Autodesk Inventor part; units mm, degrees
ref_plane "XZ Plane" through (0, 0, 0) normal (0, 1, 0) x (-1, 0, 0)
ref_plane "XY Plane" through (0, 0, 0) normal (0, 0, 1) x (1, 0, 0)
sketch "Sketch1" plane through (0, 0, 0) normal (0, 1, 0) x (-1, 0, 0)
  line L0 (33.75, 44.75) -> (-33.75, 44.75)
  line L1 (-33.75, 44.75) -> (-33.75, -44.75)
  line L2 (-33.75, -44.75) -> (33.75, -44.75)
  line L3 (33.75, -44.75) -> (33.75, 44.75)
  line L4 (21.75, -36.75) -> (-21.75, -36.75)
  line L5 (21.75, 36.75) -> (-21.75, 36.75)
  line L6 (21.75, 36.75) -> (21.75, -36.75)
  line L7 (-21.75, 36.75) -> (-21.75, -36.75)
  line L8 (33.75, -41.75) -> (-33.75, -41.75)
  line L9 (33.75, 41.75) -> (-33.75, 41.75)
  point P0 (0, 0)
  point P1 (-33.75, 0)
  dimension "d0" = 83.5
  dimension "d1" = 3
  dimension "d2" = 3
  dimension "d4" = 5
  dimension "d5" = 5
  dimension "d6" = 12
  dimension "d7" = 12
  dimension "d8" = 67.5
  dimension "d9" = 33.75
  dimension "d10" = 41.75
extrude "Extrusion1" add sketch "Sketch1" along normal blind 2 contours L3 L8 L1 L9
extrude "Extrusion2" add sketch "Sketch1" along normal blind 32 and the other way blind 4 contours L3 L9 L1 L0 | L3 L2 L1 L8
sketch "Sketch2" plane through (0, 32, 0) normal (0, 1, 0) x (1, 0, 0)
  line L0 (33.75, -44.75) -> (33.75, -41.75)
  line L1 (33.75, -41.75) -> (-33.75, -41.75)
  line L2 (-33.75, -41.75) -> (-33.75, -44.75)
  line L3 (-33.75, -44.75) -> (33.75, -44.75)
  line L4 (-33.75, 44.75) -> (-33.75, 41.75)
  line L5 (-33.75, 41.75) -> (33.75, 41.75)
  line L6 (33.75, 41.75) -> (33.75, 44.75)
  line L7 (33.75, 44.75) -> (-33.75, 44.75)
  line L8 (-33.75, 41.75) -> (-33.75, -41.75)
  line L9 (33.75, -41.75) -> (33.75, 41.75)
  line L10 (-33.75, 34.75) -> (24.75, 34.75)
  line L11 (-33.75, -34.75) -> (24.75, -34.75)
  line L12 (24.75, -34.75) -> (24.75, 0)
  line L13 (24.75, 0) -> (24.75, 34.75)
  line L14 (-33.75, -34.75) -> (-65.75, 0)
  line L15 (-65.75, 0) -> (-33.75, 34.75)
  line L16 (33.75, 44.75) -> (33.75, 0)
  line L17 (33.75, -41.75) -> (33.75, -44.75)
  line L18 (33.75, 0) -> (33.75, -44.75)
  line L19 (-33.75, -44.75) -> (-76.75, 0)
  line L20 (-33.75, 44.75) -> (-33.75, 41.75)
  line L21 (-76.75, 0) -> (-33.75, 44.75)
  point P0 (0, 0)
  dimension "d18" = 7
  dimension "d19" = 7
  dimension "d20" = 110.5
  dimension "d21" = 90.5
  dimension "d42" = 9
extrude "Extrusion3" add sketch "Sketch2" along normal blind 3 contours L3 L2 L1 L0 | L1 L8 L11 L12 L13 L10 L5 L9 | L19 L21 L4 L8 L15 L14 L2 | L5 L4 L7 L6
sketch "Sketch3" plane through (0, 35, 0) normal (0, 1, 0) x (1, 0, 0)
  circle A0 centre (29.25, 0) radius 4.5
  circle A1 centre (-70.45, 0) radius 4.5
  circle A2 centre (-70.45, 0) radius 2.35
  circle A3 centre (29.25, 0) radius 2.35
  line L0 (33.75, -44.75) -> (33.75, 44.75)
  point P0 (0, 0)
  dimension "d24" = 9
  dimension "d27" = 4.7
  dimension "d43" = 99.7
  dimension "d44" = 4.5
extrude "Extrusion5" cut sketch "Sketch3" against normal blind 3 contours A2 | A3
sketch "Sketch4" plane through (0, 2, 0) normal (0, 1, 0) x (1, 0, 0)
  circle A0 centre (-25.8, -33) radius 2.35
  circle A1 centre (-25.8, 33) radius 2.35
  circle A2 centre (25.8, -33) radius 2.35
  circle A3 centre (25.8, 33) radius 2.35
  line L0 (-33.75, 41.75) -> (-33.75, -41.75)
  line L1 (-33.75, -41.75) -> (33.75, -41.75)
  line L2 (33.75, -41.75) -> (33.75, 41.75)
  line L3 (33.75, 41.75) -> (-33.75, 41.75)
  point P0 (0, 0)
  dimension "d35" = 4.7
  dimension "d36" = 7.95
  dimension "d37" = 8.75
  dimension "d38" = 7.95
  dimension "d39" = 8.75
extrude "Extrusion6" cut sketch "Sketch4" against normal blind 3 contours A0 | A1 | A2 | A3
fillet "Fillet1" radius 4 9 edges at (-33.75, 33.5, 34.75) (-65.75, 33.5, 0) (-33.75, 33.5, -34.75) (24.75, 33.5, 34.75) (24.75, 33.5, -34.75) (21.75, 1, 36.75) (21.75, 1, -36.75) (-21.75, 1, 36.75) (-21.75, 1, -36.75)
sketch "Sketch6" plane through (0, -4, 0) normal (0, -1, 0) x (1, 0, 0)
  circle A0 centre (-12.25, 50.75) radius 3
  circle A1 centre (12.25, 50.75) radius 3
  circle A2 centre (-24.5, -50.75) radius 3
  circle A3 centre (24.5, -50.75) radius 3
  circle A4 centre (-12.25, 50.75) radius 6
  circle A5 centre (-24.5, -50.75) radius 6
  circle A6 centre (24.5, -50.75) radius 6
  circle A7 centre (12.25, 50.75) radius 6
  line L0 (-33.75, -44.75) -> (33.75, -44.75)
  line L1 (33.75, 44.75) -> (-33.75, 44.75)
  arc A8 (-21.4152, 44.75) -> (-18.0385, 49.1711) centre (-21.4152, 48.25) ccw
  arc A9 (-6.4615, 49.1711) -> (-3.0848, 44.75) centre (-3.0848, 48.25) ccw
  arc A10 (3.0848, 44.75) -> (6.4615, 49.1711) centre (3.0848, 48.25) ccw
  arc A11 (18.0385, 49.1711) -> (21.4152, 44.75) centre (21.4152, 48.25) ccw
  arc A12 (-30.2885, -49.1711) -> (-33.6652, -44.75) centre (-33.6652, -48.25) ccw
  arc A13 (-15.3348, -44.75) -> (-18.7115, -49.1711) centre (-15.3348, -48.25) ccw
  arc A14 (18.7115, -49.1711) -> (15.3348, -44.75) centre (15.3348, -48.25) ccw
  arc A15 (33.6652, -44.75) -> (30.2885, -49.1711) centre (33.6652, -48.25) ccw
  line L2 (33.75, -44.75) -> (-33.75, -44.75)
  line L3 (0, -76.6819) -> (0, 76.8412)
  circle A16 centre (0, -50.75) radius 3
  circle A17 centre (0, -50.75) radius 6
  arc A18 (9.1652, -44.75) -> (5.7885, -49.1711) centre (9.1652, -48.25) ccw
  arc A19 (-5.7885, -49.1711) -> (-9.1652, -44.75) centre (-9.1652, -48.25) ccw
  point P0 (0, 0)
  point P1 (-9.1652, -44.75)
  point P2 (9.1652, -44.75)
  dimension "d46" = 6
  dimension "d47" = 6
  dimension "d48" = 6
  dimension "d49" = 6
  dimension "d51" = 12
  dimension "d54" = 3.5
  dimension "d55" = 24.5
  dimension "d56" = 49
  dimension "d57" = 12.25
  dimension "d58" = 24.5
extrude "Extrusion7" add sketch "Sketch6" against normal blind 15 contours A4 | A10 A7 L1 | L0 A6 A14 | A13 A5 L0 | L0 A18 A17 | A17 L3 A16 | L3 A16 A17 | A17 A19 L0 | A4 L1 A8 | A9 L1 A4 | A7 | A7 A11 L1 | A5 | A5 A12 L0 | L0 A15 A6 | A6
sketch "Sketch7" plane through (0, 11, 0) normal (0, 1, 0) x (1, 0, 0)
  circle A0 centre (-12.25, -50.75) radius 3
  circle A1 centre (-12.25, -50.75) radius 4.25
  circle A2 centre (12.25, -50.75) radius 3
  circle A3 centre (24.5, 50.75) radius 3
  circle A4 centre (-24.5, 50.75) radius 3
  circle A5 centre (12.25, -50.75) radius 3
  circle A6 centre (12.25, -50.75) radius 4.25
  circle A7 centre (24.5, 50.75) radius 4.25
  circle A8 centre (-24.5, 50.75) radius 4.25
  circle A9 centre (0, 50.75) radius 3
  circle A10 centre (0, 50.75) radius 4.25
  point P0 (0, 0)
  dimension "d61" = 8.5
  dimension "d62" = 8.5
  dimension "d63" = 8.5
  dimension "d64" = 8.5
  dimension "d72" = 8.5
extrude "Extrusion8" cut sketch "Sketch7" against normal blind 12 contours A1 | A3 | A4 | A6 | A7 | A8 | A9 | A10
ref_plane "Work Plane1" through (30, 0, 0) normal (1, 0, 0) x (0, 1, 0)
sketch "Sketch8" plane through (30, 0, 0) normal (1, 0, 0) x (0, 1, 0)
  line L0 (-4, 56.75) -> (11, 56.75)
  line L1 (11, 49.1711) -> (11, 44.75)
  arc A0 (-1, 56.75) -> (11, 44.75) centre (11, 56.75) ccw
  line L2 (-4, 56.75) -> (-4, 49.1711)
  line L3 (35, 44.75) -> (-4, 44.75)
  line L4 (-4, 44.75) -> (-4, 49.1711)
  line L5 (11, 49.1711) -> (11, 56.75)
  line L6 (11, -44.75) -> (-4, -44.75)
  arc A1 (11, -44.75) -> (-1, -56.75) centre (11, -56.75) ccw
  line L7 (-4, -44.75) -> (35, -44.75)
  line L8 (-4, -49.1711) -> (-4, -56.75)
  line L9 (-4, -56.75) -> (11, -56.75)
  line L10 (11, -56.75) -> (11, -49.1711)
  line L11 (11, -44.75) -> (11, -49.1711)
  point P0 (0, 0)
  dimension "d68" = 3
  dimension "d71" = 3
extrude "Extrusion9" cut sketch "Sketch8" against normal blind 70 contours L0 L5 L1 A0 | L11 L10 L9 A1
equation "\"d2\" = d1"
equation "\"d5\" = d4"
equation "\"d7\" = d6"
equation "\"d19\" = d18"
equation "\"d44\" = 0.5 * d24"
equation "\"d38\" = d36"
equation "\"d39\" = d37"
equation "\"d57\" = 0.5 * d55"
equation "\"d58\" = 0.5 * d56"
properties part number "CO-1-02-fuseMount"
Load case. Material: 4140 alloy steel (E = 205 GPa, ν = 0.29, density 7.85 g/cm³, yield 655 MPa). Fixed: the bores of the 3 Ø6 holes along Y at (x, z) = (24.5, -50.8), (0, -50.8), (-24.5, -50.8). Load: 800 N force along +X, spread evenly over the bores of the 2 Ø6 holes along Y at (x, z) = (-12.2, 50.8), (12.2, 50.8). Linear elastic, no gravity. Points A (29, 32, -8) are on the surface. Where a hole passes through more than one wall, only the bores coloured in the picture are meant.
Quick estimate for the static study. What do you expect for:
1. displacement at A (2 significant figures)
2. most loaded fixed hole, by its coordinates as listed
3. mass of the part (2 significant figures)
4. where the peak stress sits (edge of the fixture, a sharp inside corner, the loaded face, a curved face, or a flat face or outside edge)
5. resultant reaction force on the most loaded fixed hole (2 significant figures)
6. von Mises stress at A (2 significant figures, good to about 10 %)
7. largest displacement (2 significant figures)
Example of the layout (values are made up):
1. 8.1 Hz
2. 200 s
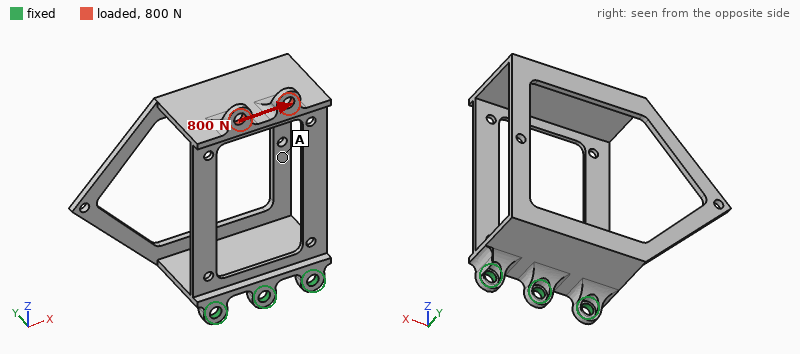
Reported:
1. 0.13 mm
2. (0, -50.8)
3. 240 g
4. a curved face
5. 1.4 kN
6. 50 MPa
7. 0.62 mm
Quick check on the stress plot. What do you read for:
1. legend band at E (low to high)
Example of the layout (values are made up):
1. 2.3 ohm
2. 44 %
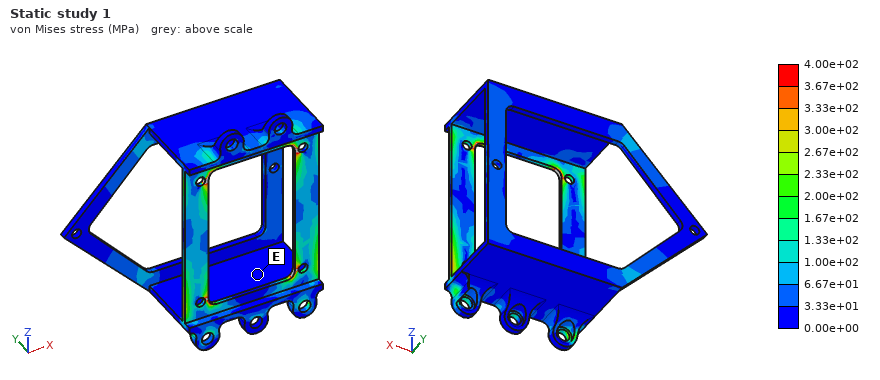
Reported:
1. 0.00e+00 to 3.33e+01 MPa
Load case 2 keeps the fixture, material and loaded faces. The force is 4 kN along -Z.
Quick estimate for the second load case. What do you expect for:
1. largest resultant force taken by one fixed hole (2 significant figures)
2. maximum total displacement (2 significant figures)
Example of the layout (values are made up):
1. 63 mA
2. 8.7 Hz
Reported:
1. 2.3 kN
2. 0.63 mm
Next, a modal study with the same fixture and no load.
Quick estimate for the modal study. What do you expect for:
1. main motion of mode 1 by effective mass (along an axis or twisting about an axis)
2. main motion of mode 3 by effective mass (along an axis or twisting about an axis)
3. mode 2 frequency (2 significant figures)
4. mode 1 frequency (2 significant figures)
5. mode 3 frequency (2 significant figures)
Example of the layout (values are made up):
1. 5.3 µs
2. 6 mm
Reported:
1. along Y
2. along X
3. 470 Hz
4. 170 Hz
5. 730 Hz
